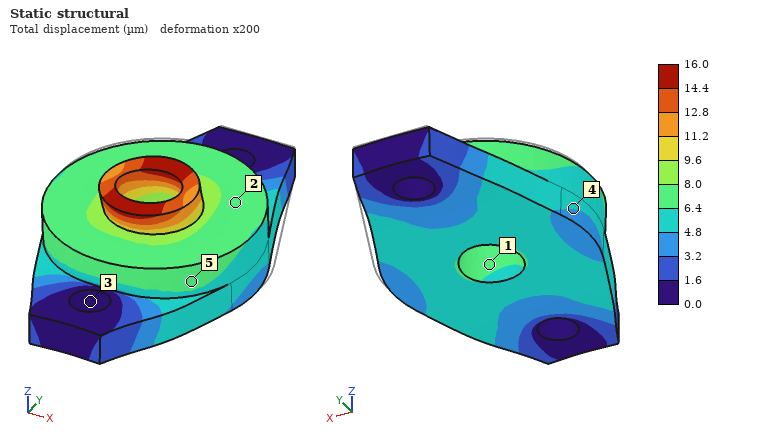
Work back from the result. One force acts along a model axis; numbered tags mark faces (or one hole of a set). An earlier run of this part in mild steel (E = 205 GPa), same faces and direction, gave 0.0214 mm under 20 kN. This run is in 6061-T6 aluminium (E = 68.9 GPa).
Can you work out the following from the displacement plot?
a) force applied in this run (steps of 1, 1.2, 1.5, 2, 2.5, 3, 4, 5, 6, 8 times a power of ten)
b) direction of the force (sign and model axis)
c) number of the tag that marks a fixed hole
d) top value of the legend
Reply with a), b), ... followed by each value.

a) 5 kN
b) -Y
c) 3
d) 16.0 µm
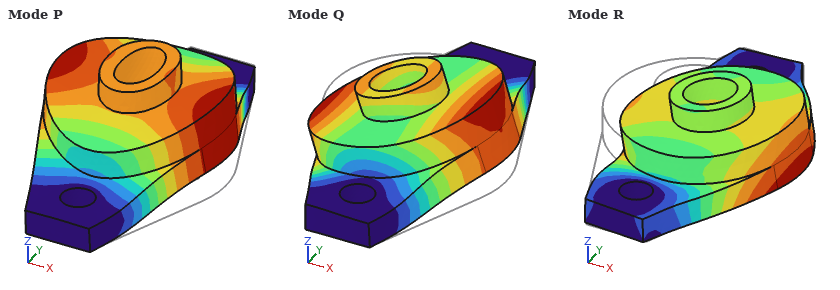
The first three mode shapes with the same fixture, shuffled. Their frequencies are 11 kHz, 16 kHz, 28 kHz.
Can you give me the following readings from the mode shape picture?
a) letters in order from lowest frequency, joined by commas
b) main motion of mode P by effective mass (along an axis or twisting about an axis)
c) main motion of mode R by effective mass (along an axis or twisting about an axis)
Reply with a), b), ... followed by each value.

a) Q, P, R
b) along Z
c) along X
